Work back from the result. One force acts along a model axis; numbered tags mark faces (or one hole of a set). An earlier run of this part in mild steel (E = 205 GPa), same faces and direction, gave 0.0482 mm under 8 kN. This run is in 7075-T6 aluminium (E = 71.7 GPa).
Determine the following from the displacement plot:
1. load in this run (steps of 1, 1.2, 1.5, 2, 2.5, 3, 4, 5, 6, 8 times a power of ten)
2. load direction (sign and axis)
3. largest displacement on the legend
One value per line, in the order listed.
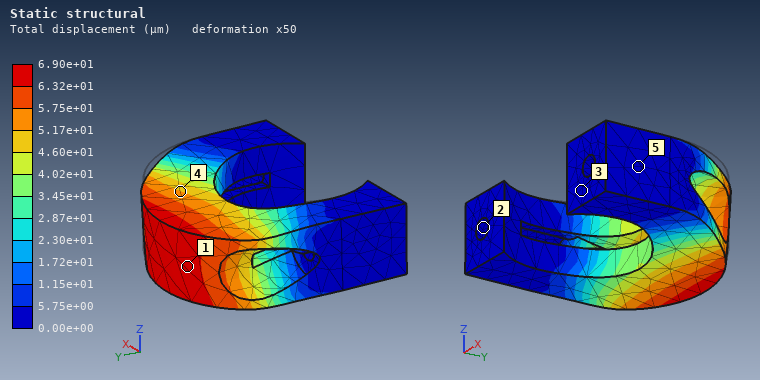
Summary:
4 kN
-Z
6.90e+01 µm
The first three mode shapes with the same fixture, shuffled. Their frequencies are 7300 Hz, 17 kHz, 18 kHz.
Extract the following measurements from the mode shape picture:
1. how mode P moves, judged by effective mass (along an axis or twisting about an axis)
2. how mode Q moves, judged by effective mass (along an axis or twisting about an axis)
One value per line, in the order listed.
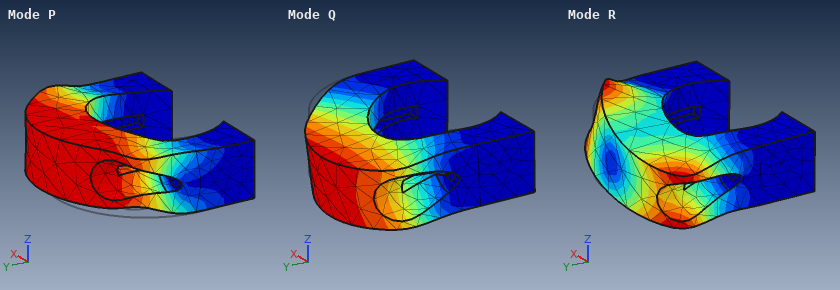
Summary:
along X
along Z
